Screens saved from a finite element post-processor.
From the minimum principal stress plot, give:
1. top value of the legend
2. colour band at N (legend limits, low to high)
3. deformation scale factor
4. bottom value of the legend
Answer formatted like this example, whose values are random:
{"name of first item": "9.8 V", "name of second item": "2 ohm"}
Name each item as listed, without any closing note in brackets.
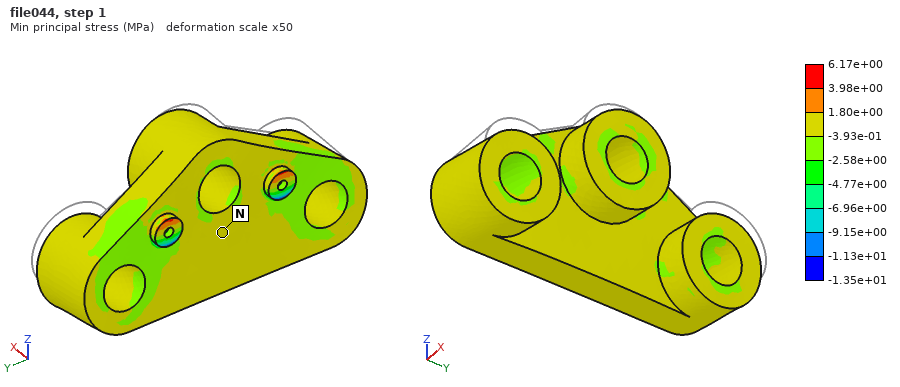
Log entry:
{"top value of the legend": "6.17e+00 MPa", "colour band at N": "-3.93e-01 to 1.80e+00 MPa", "deformation scale factor": "50", "bottom value of the legend": "-1.35e+01 MPa"}
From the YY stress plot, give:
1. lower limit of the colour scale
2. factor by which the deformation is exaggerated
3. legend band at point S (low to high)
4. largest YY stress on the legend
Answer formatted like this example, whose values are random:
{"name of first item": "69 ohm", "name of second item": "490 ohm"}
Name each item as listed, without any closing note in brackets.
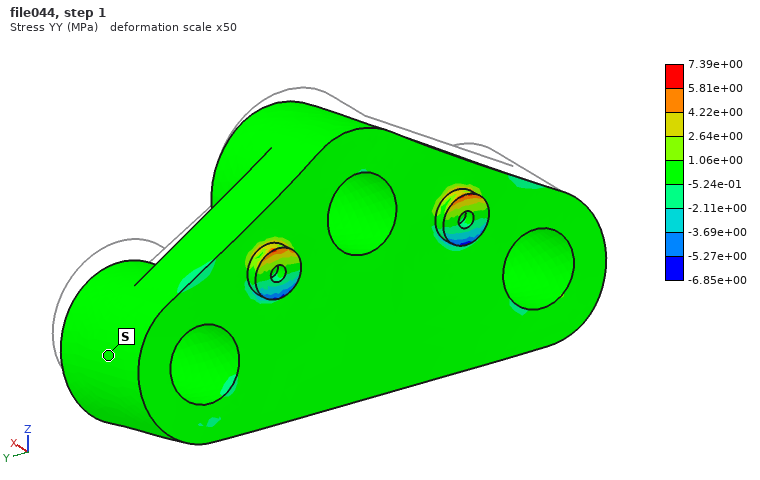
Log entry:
{"lower limit of the colour scale": "-6.85e+00 MPa", "factor by which the deformation is exaggerated": "50", "legend band at point S": "-5.24e-01 to 1.06e+00 MPa", "largest YY stress on the legend": "7.39e+00 MPa"}
